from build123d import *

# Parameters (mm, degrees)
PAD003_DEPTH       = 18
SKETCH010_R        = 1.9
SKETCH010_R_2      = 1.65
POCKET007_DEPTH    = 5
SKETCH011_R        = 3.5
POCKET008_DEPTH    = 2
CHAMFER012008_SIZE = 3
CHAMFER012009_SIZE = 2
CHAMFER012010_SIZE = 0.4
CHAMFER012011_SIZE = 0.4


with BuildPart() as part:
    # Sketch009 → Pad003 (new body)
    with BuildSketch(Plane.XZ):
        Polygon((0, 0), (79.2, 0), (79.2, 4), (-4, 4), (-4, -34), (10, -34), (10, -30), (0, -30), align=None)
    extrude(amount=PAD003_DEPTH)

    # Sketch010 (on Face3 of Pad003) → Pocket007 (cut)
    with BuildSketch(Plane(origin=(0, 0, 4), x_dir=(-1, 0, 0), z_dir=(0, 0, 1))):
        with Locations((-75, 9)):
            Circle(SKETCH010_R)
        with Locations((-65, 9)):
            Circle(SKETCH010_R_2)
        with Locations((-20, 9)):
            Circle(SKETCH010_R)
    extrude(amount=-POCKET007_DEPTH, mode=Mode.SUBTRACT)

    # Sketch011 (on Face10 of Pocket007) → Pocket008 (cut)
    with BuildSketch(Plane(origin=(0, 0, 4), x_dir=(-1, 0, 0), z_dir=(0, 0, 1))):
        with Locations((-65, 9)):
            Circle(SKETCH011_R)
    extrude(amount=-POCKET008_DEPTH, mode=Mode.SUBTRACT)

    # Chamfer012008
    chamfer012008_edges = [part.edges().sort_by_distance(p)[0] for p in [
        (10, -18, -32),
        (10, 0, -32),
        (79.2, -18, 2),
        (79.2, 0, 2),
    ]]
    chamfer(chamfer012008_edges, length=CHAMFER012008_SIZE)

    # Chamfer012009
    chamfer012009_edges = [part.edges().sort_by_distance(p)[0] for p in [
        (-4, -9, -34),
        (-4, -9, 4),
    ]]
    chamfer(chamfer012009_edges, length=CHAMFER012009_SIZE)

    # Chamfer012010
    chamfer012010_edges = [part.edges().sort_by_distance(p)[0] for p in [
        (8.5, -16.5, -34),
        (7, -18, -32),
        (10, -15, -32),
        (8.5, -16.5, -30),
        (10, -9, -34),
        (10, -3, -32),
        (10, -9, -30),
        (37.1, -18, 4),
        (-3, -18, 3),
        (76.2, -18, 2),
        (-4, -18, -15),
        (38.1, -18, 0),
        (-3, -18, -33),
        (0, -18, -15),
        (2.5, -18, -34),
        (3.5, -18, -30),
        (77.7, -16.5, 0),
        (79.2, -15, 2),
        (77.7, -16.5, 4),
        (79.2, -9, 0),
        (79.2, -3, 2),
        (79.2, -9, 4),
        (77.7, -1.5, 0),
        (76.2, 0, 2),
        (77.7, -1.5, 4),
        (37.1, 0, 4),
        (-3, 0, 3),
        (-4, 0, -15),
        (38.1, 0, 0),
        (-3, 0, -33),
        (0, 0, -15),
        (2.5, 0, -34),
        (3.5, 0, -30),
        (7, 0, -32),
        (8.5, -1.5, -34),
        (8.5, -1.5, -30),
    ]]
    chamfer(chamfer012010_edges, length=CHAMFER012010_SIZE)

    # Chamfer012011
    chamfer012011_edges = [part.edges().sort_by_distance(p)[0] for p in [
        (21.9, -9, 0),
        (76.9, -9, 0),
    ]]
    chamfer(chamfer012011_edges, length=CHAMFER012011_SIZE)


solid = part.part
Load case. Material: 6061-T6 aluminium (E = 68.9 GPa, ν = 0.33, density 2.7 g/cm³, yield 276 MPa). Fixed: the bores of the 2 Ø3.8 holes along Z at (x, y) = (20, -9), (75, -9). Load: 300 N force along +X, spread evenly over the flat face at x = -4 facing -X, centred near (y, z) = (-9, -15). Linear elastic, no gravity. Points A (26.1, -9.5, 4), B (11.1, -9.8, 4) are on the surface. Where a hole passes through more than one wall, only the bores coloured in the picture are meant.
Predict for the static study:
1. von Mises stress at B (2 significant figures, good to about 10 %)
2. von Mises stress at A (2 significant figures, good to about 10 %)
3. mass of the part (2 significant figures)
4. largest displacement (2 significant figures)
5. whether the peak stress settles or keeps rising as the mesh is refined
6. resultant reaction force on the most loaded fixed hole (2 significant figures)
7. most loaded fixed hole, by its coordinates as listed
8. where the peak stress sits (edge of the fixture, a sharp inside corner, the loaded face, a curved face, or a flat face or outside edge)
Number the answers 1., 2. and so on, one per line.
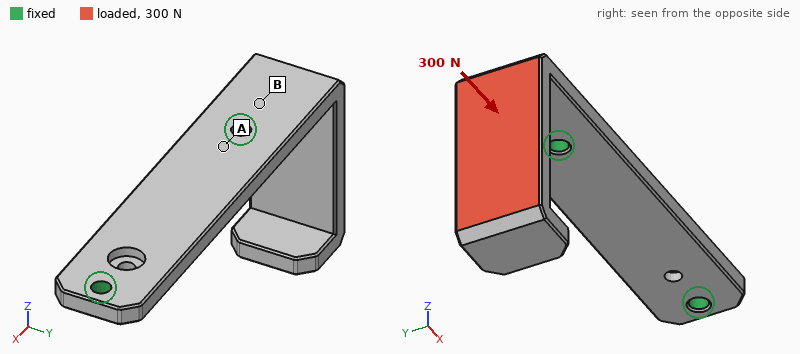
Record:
1. 94 MPa
2. 17 MPa
3. 24 g
4. 0.83 mm
5. keeps rising
6. 280 N
7. (20, -9)
8. edge of the fixture
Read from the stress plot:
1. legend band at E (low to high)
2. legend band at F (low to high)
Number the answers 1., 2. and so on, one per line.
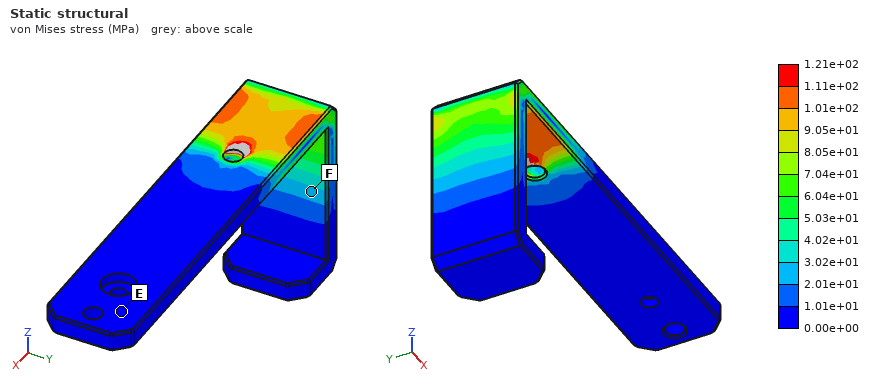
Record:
1. 0.00e+00 to 1.01e+01 MPa
2. 2.01e+01 to 3.02e+01 MPa
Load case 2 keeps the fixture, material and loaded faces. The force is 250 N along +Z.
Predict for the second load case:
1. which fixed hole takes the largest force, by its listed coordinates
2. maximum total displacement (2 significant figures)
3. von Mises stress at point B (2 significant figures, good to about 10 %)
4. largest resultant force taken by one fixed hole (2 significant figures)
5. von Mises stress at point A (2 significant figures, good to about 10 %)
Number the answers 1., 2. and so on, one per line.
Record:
1. (20, -9)
2. 0.45 mm
3. 73 MPa
4. 260 N
5. 14 MPa
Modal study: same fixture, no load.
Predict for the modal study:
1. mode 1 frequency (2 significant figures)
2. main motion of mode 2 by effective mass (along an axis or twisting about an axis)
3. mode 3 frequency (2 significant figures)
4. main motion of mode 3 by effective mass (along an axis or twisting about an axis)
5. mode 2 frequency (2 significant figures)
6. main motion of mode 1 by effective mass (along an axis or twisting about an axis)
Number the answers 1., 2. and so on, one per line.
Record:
1. 1000 Hz
2. along Y
3. 3100 Hz
4. along Z
5. 1400 Hz
6. along X
